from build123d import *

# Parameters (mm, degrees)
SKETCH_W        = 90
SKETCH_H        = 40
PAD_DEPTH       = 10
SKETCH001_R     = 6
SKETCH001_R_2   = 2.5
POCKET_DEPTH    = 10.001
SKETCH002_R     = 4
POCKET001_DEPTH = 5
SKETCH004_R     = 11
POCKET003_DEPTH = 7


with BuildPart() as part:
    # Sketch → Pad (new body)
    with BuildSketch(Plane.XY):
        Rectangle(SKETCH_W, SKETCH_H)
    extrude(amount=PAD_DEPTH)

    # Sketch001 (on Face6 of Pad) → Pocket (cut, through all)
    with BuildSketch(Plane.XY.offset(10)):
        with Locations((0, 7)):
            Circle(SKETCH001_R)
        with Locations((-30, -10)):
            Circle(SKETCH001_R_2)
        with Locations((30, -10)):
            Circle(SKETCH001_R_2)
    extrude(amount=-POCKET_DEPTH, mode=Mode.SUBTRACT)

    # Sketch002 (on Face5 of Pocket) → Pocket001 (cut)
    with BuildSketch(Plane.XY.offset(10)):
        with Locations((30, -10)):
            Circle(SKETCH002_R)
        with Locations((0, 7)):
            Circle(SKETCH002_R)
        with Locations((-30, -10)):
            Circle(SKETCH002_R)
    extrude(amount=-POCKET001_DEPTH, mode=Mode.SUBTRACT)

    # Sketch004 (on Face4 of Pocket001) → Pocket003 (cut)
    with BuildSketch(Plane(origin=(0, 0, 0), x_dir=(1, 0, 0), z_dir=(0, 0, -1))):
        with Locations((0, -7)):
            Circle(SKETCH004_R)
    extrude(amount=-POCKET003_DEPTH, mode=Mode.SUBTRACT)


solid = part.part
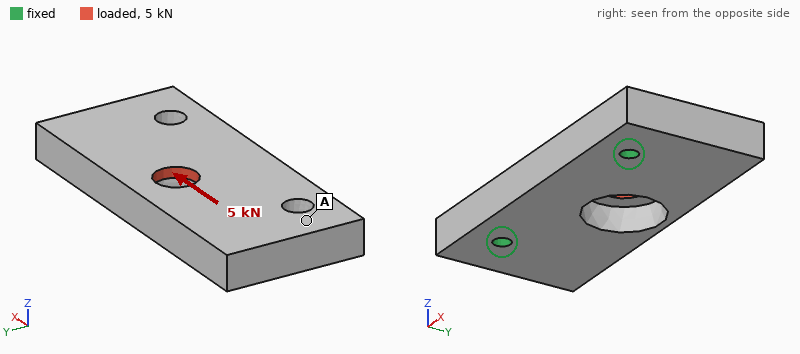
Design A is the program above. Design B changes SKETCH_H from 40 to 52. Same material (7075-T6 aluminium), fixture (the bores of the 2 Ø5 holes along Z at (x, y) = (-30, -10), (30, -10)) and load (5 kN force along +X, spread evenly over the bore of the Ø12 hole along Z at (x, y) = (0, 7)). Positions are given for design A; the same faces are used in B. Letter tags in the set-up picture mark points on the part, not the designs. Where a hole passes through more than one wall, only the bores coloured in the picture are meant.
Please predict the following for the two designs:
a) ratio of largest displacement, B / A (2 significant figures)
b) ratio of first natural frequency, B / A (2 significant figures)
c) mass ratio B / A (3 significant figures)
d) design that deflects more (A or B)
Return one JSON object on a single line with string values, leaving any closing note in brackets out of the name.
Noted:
{"ratio of largest displacement, B / A": "0.90", "ratio of first natural frequency, B / A": "0.73", "mass ratio B / A": "1.33", "design that deflects more": "A"}
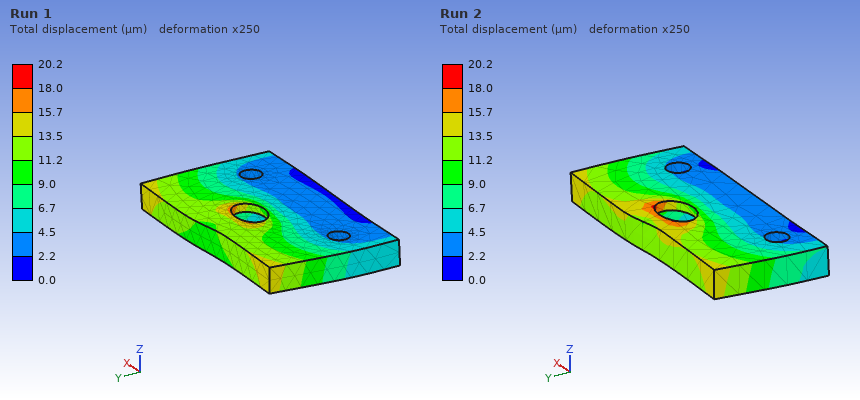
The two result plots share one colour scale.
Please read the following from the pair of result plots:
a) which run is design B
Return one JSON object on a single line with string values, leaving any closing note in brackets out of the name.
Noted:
{"which run is design B": "Run 1"}
